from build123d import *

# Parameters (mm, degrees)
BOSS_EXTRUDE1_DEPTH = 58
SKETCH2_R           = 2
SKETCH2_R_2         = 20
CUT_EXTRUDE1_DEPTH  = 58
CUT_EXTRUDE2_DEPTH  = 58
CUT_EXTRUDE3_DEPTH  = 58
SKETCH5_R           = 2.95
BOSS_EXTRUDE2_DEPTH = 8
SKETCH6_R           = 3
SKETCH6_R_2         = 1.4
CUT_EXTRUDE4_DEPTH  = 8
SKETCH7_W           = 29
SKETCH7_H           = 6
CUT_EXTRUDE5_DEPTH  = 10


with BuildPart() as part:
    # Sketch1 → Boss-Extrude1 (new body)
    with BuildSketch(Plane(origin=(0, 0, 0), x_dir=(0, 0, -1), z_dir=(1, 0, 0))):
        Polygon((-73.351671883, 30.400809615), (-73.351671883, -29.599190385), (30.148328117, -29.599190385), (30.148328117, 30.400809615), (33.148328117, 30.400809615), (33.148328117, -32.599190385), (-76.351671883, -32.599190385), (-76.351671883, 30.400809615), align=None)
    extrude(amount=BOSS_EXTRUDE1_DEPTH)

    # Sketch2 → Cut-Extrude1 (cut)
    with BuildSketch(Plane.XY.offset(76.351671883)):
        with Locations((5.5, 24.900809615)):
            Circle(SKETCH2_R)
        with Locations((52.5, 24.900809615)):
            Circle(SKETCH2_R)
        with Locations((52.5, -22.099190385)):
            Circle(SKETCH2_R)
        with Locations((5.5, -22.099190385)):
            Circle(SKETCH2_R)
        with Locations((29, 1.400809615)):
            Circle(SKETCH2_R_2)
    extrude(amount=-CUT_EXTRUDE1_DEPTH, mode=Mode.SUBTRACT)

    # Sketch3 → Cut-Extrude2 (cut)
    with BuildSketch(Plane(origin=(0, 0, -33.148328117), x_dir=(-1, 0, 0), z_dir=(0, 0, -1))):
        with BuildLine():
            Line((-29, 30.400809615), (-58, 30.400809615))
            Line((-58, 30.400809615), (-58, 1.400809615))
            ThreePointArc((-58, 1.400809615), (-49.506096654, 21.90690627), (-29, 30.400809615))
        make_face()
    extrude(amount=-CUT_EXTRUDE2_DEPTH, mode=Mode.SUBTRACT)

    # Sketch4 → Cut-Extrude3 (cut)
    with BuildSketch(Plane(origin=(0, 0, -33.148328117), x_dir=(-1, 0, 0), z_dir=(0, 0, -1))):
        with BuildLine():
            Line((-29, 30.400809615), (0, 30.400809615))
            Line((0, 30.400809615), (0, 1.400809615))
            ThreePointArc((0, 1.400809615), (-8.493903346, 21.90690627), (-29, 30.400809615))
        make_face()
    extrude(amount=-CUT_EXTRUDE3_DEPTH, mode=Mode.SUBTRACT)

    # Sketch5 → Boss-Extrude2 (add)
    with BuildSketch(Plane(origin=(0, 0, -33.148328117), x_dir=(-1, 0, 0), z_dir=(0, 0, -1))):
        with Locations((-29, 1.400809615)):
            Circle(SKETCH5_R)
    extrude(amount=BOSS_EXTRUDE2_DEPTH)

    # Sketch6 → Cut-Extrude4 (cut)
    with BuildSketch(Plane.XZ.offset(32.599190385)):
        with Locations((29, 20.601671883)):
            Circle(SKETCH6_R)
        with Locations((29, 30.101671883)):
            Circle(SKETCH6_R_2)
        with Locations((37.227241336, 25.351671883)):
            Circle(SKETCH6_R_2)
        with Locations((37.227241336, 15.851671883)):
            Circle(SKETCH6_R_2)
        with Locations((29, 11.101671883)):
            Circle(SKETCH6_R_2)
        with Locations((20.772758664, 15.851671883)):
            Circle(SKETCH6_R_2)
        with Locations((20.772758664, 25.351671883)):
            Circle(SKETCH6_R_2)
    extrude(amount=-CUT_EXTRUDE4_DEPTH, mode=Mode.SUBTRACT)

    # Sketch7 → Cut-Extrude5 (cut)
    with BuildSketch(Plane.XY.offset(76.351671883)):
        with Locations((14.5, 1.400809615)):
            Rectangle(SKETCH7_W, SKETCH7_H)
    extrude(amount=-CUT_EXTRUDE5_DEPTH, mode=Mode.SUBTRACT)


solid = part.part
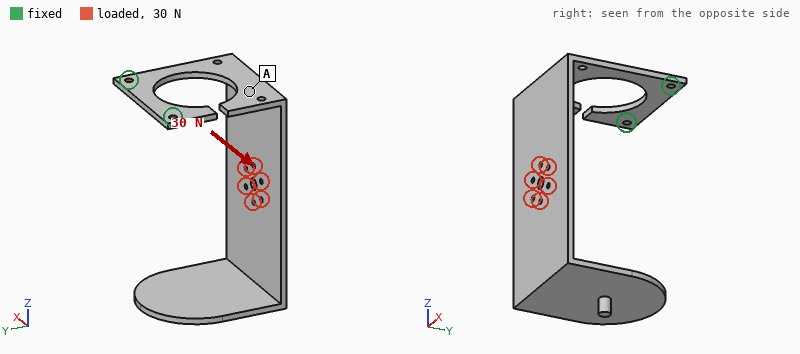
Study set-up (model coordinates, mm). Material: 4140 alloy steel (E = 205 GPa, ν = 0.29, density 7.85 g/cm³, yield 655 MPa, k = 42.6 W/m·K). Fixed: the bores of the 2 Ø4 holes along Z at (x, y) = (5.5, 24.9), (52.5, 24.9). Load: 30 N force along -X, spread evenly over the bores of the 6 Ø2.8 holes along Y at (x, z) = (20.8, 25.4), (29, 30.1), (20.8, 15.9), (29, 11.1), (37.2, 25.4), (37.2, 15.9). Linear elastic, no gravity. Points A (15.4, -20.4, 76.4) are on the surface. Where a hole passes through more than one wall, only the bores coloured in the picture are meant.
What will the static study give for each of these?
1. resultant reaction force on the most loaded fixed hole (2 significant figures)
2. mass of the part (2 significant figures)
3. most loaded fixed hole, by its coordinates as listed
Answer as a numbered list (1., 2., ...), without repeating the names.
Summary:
1. 35 N
2. 270 g
3. (52.5, 24.9)
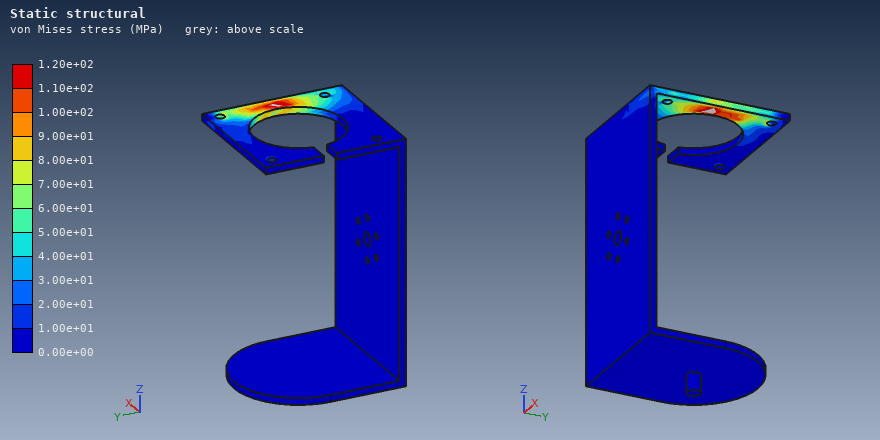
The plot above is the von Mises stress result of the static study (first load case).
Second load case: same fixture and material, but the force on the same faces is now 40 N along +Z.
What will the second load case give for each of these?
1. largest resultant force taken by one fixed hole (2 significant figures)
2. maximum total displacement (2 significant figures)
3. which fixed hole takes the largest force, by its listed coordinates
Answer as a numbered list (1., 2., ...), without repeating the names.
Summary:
1. 40 N
2. 1.6 mm
3. (52.5, 24.9)
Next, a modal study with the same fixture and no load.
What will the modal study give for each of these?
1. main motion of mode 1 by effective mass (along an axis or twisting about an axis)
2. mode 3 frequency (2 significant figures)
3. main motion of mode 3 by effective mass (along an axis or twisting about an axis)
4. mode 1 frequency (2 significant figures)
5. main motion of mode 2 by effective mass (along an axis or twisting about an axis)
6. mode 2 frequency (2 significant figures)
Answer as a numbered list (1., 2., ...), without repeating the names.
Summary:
1. along Y
2. 180 Hz
3. along Z
4. 39 Hz
5. along X
6. 48 Hz
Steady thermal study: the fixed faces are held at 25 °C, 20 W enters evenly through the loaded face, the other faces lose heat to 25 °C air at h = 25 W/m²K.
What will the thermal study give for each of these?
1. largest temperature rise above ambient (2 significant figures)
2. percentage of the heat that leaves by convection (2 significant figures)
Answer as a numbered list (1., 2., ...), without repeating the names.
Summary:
1. 74 K
2. 97 %
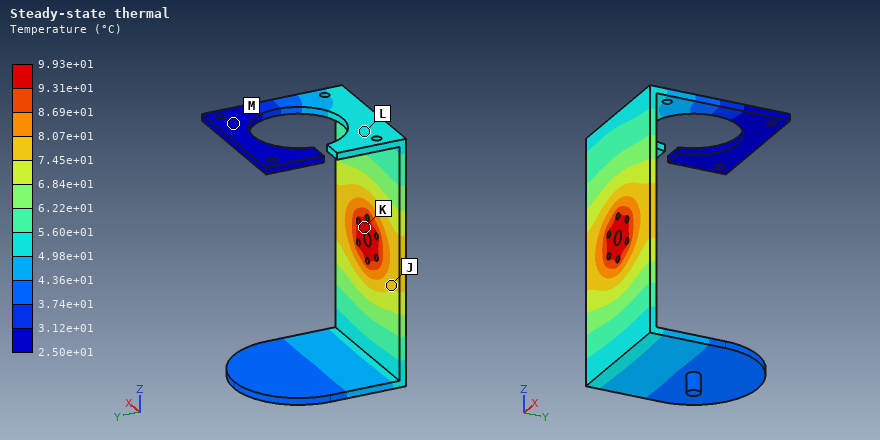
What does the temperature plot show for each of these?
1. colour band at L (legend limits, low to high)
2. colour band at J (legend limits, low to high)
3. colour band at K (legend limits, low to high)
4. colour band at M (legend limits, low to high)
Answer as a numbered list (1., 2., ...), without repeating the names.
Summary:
1. 4.98e+01 to 5.60e+01 °C
2. 7.45e+01 to 8.07e+01 °C
3. 9.31e+01 to 9.93e+01 °C
4. 2.50e+01 to 3.12e+01 °C
